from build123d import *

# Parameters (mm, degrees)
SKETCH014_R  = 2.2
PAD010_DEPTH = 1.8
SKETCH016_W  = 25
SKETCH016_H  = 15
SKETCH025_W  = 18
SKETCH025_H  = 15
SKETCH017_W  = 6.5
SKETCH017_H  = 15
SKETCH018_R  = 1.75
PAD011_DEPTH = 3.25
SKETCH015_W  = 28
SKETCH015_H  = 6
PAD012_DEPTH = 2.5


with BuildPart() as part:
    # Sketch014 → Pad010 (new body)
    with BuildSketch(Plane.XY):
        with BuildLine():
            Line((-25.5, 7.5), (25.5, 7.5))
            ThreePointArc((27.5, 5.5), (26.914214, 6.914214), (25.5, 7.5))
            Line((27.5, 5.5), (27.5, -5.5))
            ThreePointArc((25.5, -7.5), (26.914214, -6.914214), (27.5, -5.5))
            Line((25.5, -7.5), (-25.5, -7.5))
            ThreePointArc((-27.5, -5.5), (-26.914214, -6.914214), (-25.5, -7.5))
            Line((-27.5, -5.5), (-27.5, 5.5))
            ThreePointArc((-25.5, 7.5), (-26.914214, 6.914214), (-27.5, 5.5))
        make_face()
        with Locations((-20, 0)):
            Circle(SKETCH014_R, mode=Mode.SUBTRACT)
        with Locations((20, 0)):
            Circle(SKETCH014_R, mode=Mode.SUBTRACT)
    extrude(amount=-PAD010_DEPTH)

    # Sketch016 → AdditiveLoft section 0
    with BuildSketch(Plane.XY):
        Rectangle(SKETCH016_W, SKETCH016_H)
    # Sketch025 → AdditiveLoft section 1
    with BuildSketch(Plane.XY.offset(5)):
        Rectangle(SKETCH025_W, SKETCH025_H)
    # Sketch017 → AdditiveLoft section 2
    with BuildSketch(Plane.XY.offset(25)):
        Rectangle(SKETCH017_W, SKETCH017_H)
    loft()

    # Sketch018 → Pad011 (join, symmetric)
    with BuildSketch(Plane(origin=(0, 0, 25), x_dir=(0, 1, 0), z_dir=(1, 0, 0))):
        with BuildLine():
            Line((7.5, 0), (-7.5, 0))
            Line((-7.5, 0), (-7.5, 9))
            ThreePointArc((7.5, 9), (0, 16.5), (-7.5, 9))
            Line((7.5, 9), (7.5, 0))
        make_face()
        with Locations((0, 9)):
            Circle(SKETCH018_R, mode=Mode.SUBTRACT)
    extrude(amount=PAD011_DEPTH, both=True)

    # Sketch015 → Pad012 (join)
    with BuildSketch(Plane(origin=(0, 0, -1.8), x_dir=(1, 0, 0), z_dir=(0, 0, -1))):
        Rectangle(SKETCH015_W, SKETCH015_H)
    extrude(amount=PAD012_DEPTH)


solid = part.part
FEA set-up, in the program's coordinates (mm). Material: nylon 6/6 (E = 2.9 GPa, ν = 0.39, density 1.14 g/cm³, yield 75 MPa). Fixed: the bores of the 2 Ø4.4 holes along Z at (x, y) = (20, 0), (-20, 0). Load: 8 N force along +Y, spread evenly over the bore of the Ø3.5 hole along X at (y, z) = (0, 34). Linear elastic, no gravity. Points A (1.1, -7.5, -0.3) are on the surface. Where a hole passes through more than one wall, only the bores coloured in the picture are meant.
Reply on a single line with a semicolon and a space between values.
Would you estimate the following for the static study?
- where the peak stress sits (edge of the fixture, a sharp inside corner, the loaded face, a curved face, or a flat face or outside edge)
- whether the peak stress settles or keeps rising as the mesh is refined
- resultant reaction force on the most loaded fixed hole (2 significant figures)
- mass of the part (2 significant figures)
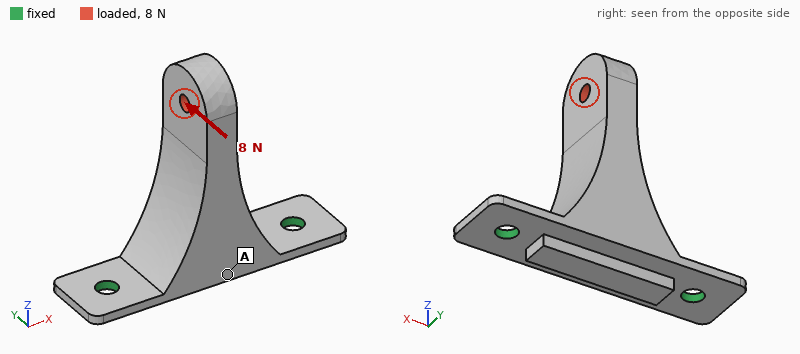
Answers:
edge of the fixture; keeps rising; 4.0 N; 9.1 g
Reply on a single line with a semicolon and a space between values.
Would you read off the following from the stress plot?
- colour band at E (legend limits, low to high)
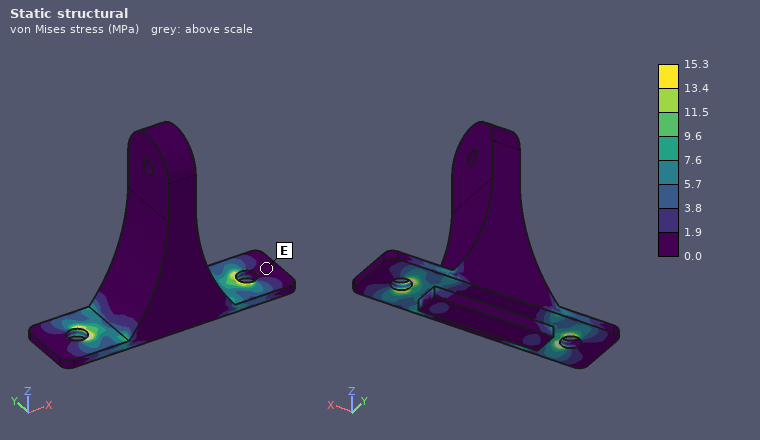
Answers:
0.0 to 1.9 MPa
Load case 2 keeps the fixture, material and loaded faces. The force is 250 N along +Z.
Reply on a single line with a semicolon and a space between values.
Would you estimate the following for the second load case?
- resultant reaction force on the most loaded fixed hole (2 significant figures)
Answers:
130 N
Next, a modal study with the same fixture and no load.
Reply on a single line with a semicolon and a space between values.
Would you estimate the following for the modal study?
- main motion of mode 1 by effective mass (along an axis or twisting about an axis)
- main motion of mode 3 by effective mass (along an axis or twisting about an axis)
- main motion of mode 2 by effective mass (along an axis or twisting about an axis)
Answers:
along Y; along Z; along X
